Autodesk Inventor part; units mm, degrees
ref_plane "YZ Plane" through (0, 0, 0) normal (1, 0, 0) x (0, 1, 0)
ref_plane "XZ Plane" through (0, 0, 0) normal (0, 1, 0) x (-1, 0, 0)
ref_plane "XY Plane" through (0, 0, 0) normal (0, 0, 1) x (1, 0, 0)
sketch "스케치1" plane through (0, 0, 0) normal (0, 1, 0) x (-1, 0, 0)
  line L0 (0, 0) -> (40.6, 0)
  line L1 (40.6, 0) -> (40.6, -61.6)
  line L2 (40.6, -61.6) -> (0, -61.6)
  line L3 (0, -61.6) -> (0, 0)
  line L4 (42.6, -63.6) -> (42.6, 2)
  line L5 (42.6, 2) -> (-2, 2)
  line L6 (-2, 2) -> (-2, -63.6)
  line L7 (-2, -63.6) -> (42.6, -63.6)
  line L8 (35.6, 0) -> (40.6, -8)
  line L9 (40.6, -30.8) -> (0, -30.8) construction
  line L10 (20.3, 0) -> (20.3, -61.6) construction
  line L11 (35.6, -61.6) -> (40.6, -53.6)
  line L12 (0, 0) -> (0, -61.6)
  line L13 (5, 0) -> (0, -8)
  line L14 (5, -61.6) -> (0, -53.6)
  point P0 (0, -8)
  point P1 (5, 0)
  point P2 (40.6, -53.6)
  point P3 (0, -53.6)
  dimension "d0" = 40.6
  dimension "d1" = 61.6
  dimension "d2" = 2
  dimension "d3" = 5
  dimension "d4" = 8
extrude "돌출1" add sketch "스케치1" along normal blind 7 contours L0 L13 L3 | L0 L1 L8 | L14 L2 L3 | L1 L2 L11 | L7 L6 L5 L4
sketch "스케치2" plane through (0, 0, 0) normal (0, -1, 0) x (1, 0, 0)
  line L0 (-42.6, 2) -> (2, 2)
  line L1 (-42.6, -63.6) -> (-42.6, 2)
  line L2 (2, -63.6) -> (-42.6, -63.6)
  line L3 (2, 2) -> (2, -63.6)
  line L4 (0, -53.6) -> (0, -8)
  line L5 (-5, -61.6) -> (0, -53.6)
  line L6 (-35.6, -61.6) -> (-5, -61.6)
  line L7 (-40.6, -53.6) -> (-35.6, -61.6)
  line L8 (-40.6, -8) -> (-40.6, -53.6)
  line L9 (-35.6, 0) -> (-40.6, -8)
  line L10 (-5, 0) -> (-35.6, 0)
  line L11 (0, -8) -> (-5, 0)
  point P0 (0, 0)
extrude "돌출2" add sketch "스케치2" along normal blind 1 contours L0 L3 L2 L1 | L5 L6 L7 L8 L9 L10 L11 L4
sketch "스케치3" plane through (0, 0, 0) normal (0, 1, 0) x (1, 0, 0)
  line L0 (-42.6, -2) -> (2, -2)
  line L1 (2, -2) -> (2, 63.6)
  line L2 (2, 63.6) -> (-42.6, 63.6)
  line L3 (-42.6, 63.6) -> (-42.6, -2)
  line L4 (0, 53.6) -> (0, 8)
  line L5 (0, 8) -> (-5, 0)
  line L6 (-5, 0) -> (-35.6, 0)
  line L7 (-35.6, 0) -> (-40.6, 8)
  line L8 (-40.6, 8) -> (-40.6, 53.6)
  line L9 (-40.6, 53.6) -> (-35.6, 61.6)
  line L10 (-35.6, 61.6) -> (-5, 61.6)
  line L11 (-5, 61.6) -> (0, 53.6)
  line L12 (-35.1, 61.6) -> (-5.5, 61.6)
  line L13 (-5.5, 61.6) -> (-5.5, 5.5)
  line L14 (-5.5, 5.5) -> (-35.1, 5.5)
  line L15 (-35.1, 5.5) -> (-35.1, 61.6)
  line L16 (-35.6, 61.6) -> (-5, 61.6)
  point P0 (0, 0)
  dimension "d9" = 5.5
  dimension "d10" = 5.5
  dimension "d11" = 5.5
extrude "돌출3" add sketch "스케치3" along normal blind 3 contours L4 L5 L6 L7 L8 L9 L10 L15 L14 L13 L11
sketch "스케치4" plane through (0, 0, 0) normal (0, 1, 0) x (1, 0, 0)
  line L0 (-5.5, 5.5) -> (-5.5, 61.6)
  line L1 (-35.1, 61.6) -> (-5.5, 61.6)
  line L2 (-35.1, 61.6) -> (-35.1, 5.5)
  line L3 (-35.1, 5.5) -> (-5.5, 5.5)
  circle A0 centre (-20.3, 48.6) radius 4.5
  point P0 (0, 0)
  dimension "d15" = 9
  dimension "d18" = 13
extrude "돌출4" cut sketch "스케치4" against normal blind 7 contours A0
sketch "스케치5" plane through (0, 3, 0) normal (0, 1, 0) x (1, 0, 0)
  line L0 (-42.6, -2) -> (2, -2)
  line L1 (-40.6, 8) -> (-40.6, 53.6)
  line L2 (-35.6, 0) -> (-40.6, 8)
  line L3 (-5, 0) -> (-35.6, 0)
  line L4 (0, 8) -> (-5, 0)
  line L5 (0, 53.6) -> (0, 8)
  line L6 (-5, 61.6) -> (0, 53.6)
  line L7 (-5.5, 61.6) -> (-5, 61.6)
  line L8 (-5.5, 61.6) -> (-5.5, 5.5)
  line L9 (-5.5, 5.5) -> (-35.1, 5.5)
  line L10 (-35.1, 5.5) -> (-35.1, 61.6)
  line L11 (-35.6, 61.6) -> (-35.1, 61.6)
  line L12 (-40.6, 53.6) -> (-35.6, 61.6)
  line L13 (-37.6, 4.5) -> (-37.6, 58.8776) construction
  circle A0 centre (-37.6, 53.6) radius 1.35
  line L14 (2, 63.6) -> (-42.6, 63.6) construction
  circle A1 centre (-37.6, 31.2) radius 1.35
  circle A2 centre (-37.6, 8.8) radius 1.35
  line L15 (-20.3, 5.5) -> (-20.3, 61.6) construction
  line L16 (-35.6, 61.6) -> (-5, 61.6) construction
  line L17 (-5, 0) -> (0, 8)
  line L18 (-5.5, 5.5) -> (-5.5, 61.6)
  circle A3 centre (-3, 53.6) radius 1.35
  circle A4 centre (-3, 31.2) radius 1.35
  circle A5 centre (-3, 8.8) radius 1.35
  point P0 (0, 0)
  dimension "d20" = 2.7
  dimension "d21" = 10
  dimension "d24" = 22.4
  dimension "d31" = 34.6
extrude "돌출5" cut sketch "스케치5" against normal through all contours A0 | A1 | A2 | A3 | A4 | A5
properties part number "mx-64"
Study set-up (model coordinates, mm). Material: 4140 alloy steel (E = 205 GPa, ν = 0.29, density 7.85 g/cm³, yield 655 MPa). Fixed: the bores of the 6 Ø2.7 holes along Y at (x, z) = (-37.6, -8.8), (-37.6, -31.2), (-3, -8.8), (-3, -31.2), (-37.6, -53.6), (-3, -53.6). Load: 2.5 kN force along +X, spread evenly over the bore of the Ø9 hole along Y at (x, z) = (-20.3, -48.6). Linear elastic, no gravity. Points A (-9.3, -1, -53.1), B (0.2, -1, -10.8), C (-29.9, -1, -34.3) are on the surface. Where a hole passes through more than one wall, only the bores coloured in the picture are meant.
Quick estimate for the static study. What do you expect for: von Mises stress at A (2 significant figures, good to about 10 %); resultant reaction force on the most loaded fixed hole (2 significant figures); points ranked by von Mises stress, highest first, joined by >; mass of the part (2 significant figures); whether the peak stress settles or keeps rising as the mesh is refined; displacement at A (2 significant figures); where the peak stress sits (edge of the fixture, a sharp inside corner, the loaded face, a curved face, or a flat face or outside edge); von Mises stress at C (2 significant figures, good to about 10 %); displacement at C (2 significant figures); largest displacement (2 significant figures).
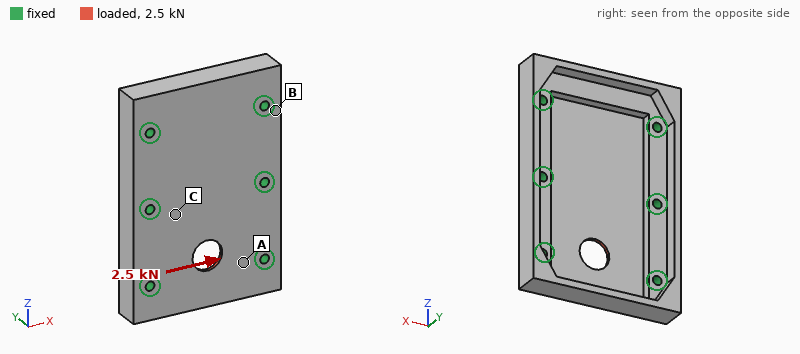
71 MPa
880 N
A > C > B
67 g
keeps rising
2.4 µm
a sharp inside corner
25 MPa
1.4 µm
5.6 µm
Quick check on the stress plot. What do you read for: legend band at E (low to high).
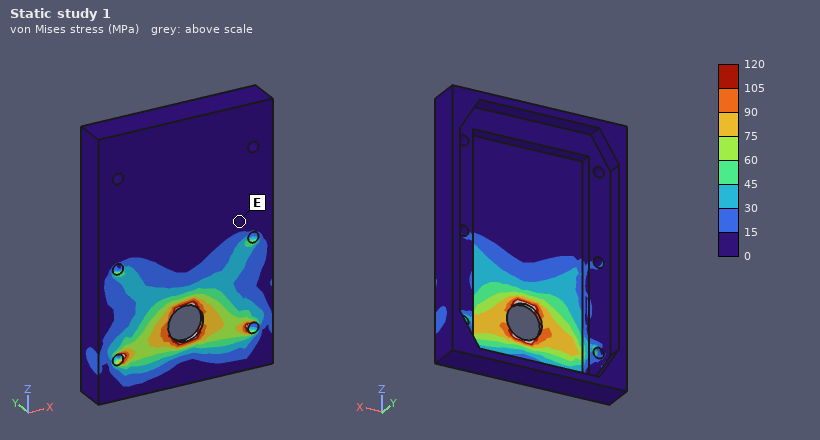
0 to 15 MPa
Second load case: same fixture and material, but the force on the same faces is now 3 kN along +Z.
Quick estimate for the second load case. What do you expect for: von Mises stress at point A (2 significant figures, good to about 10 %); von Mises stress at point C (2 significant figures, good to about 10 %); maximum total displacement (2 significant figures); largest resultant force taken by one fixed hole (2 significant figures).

66 MPa
52 MPa
12 µm
790 N
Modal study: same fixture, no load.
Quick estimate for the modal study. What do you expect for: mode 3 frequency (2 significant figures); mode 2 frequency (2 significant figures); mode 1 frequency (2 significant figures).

12 kHz
8700 Hz
6400 Hz
